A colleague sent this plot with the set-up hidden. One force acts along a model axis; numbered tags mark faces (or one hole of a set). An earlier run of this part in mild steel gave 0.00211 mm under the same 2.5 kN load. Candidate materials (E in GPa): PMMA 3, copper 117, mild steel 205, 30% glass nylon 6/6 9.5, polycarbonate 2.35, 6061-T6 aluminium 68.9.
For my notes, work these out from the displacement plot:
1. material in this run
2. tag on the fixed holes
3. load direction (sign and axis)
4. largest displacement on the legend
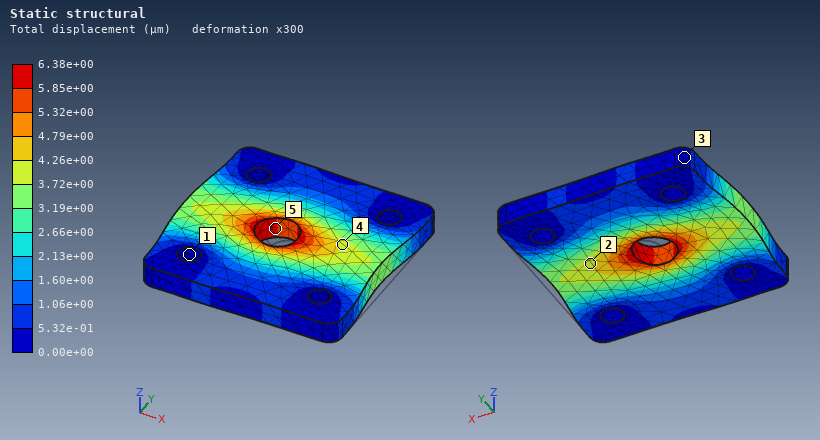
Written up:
6061-T6 aluminium
1
-X
6.38e+00 µm
